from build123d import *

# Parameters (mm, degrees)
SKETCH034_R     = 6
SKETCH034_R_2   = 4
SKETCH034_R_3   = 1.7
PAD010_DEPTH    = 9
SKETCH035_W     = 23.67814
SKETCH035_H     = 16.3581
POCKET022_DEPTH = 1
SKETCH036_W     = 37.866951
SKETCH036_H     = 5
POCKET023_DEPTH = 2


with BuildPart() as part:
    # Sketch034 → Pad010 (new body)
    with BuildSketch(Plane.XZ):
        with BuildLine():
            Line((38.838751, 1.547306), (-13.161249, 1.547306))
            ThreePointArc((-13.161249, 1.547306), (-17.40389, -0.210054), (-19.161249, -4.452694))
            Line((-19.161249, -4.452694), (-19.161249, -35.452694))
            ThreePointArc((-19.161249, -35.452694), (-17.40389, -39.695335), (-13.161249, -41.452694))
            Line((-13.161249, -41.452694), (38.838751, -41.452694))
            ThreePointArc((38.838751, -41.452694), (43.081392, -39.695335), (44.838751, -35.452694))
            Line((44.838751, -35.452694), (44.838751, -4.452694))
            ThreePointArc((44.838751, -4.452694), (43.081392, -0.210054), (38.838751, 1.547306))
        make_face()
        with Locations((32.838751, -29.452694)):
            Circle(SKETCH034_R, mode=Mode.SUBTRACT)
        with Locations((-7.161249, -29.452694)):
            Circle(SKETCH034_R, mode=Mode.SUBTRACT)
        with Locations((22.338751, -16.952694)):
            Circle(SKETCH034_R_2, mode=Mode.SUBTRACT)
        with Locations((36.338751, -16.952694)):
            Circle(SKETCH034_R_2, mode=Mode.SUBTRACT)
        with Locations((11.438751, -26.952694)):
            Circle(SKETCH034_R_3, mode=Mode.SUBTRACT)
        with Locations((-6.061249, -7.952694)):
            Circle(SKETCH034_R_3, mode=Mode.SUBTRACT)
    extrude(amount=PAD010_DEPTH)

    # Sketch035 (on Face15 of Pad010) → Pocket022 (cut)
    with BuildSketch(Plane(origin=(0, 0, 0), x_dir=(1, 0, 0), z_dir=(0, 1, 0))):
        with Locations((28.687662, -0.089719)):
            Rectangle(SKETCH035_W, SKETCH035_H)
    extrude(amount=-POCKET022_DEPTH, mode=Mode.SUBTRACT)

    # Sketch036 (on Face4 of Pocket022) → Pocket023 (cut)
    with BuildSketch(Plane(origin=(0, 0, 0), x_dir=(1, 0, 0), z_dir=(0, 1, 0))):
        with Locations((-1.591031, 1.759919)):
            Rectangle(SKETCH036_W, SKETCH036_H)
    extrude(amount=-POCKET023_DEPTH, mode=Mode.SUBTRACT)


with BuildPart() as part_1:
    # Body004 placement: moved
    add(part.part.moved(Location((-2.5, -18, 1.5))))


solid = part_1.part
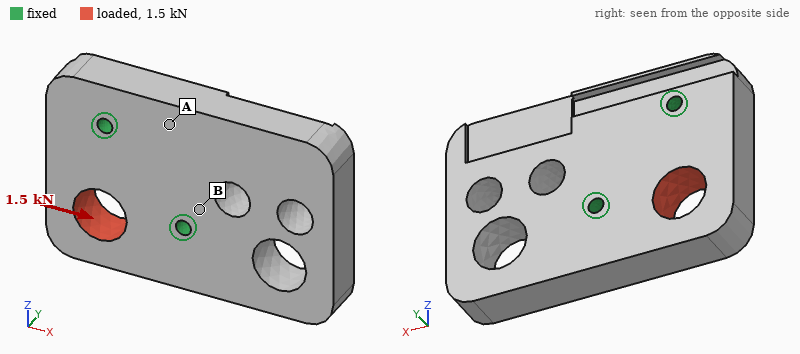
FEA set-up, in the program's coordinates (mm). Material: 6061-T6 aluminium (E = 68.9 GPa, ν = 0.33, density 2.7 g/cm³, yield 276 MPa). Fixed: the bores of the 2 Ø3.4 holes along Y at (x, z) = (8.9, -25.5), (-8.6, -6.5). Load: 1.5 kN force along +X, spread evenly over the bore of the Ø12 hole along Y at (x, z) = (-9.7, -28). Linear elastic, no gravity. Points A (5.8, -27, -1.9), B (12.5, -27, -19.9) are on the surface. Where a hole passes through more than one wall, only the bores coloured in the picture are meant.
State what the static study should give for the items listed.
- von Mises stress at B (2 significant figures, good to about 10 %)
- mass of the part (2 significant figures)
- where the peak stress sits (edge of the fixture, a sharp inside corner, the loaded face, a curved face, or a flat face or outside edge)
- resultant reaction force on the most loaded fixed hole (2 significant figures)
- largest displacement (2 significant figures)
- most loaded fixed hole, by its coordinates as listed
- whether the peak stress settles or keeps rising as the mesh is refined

4.7 MPa
56 g
edge of the fixture
1.4 kN
5.7 µm
(8.9, -25.5)
keeps rising
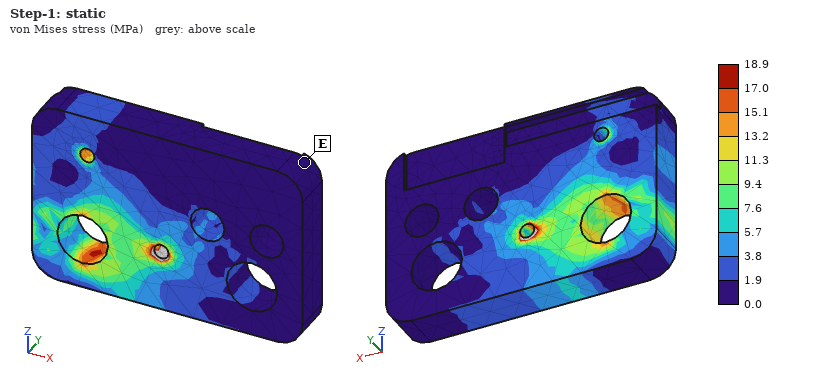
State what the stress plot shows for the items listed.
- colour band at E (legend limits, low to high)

0.0 to 1.9 MPa
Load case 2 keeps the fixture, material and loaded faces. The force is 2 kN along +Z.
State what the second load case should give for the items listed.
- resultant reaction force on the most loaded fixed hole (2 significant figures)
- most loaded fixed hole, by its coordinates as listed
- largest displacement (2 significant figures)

1.6 kN
(-8.6, -6.5)
7.3 µm
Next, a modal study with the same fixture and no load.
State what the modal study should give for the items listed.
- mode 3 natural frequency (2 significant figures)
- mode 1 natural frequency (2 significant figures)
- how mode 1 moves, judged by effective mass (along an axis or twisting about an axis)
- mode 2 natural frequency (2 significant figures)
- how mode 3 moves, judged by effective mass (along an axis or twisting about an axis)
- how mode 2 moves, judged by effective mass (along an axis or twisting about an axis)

11 kHz
4600 Hz
along Y
8100 Hz
along Y
twisting about X
